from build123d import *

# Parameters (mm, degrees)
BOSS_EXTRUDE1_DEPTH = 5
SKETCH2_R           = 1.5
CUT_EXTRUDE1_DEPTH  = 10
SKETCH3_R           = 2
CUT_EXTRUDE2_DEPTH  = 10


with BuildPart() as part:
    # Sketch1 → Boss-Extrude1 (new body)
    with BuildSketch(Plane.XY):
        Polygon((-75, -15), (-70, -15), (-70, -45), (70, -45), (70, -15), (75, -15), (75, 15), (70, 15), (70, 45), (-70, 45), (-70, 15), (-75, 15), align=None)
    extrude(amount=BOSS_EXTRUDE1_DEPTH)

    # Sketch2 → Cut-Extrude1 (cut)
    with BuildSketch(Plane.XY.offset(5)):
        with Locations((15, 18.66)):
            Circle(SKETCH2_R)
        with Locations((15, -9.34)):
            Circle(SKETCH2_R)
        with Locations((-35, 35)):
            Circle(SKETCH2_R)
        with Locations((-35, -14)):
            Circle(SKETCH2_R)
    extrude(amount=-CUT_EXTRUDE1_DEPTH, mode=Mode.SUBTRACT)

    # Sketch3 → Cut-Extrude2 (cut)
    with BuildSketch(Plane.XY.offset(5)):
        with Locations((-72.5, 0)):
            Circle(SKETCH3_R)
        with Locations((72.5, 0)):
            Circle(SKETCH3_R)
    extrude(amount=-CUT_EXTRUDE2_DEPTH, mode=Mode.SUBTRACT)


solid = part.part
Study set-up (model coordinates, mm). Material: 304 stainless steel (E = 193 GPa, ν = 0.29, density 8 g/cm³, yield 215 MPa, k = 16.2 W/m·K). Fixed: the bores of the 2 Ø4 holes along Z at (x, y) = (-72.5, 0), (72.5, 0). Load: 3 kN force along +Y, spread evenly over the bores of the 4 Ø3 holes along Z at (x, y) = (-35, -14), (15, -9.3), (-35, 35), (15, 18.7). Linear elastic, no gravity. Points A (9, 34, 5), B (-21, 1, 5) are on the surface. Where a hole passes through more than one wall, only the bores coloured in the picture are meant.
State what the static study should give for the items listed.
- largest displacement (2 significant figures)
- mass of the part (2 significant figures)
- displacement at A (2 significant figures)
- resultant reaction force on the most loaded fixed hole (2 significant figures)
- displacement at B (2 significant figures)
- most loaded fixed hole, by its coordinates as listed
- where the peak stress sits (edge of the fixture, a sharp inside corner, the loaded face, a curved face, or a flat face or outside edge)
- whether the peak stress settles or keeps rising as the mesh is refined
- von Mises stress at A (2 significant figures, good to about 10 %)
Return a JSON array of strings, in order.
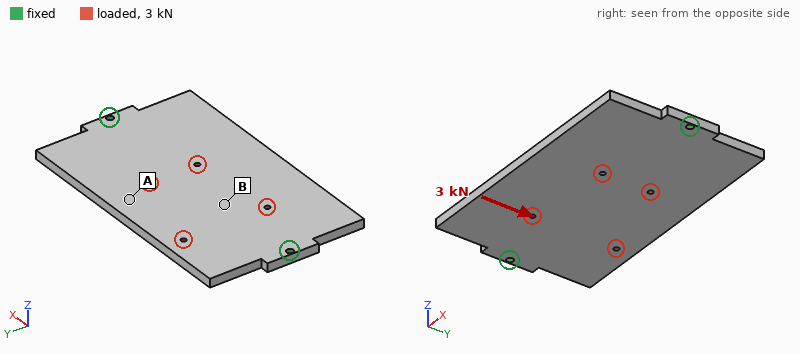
["6.5 µm", "510 g", "6.0 µm", "1.7 kN", "5.8 µm", "(-72.5, 0)", "edge of the fixture", "keeps rising", "8.6 MPa"]
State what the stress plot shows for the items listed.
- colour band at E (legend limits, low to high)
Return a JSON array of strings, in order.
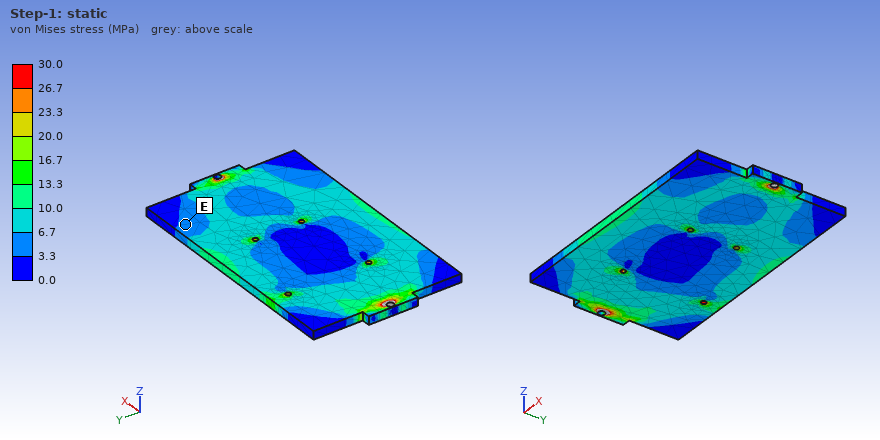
["3.3 to 6.7 MPa"]
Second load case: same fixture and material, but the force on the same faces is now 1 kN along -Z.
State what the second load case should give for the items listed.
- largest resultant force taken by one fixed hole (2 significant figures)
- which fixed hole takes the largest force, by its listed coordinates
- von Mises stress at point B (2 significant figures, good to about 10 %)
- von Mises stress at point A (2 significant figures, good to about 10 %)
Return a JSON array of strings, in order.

["580 N", "(-72.5, 0)", "31 MPa", "36 MPa"]
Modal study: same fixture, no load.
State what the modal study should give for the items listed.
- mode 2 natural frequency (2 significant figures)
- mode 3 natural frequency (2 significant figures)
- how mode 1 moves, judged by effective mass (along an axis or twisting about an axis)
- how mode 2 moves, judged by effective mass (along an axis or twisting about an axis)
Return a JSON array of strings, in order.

["790 Hz", "1800 Hz", "twisting about X", "along Z"]
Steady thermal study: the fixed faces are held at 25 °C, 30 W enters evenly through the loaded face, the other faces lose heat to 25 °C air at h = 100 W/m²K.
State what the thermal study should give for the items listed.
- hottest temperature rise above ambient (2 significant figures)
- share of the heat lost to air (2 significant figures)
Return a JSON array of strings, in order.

["50 K", "96 %"]
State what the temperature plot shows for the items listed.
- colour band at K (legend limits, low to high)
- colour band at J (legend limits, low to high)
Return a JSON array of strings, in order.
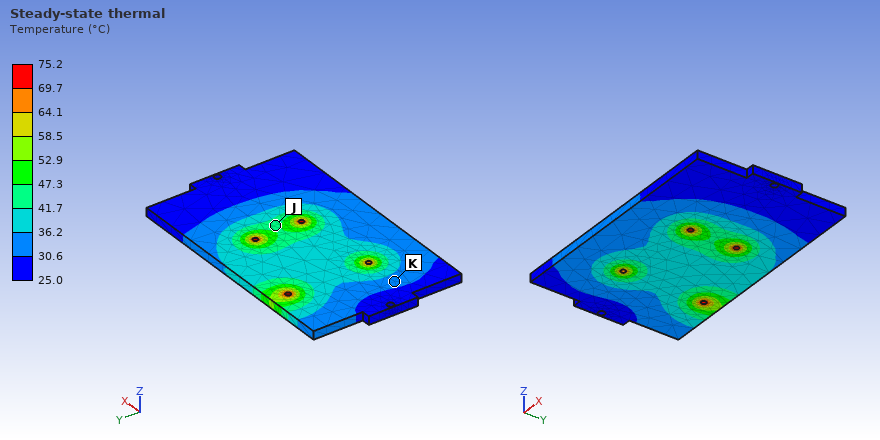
["30.6 to 36.2 °C", "41.7 to 47.3 °C"]
